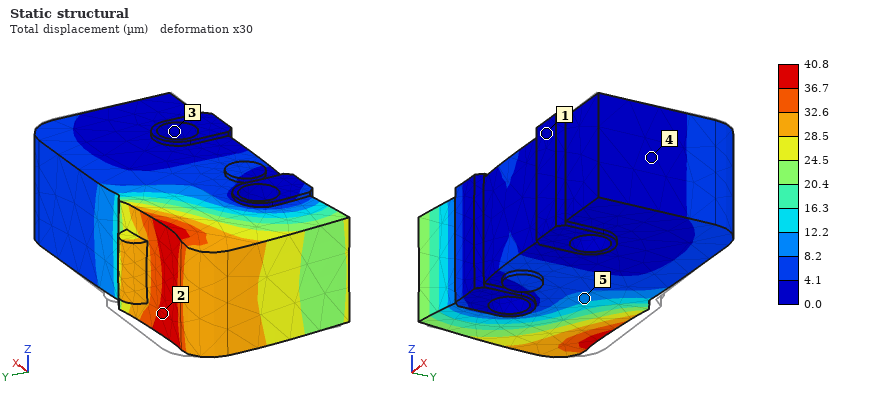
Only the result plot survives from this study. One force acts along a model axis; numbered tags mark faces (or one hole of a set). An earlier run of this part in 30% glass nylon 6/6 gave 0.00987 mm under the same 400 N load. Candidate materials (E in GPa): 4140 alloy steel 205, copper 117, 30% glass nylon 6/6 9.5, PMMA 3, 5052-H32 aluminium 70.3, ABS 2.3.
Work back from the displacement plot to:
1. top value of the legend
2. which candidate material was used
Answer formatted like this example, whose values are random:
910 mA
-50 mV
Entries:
40.8 µm
ABS
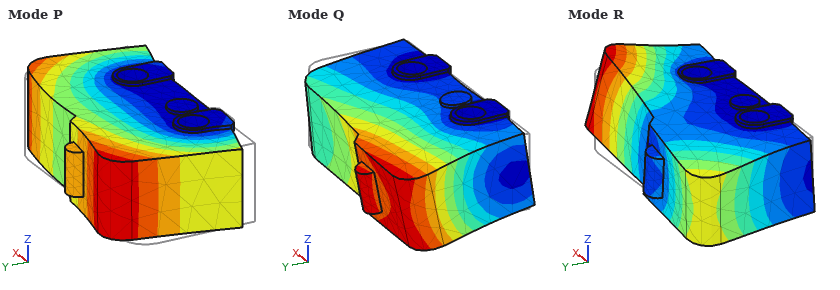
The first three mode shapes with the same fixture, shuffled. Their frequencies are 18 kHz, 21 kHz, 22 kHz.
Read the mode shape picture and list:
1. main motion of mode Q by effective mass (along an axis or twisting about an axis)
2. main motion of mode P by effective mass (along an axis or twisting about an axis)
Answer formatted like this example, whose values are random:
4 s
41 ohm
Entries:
along Z
along X
